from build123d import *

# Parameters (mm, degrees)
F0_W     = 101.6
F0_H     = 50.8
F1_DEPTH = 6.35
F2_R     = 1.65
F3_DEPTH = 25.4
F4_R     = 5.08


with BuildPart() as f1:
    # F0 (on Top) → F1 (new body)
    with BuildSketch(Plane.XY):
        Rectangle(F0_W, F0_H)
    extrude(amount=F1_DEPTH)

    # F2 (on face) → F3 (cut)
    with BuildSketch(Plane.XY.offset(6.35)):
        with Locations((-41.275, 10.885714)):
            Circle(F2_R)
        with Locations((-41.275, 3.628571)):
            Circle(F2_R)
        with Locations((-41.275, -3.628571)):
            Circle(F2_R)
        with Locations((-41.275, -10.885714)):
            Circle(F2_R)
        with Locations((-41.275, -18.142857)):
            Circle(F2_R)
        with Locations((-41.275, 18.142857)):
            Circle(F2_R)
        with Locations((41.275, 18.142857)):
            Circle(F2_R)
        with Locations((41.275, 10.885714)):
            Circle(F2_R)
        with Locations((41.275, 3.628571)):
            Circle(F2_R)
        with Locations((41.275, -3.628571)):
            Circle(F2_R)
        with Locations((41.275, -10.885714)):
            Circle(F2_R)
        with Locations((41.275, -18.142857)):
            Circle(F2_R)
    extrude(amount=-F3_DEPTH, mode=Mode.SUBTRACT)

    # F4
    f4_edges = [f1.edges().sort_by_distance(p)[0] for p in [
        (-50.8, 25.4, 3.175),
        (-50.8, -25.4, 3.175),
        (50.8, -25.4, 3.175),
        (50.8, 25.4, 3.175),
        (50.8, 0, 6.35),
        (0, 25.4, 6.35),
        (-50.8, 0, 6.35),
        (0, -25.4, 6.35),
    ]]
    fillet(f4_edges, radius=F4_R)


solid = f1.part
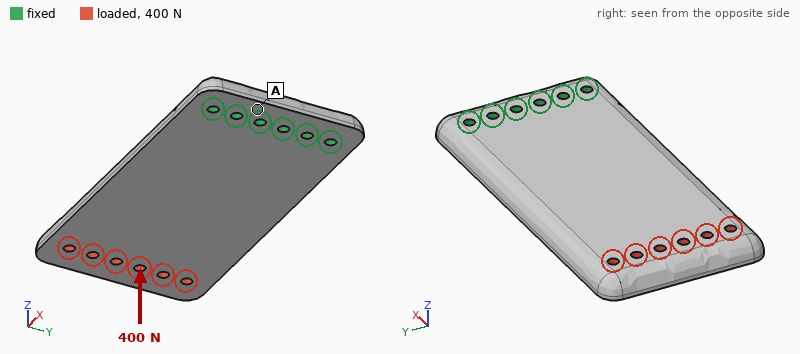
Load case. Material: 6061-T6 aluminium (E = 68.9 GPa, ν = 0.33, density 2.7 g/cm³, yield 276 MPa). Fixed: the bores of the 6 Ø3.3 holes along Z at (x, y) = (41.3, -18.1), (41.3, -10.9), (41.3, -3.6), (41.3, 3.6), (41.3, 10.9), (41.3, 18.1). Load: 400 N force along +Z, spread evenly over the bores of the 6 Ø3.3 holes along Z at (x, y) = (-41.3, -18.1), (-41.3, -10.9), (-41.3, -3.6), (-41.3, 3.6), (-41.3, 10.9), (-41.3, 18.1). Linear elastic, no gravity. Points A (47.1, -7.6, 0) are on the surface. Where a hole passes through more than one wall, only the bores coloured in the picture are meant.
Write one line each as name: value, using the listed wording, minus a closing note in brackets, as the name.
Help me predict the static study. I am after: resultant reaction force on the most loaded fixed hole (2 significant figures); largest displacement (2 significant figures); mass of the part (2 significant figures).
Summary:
resultant reaction force on the most loaded fixed hole: 220 N
largest displacement: 1.2 mm
mass of the part: 82 g
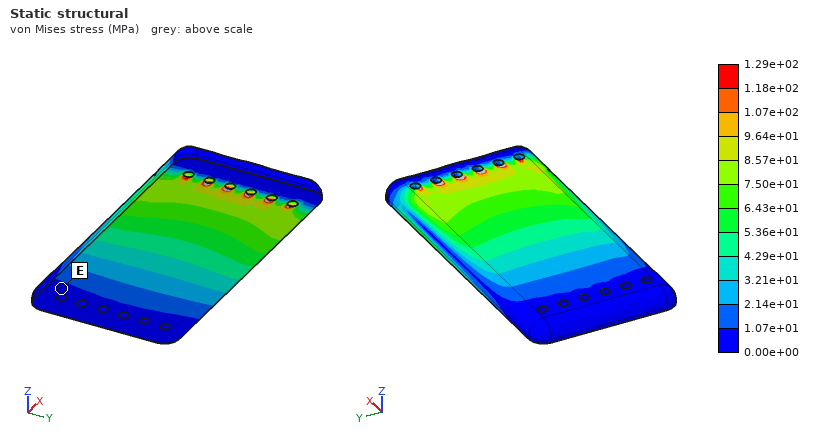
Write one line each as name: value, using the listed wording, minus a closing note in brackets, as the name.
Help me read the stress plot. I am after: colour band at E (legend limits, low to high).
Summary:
colour band at E: 0.00e+00 to 1.07e+01 MPa
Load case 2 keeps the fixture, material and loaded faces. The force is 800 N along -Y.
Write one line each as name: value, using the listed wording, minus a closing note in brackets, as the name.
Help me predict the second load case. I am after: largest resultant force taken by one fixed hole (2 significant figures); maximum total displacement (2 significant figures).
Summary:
largest resultant force taken by one fixed hole: 1.4 kN
maximum total displacement: 55 µm
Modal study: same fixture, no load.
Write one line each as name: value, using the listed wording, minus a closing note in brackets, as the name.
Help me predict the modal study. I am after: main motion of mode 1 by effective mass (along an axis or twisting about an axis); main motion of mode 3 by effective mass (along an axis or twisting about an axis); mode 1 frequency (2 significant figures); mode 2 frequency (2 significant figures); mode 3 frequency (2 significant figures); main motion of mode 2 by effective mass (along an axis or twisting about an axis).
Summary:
main motion of mode 1 by effective mass: along Z
main motion of mode 3 by effective mass: along Z
mode 1 frequency: 650 Hz
mode 2 frequency: 2400 Hz
mode 3 frequency: 3900 Hz
main motion of mode 2 by effective mass: twisting about X
